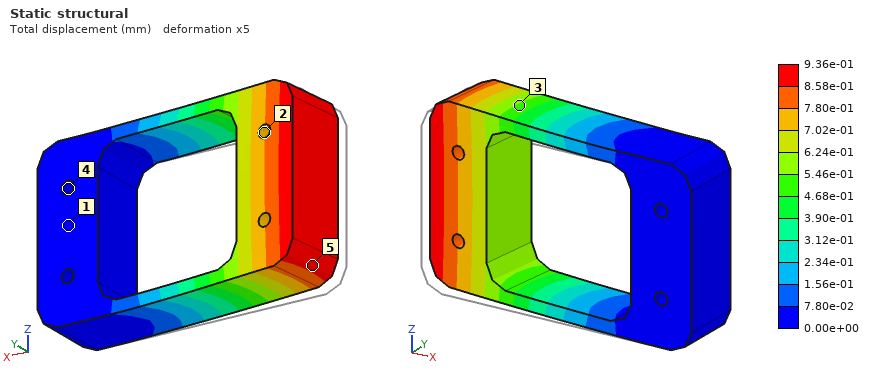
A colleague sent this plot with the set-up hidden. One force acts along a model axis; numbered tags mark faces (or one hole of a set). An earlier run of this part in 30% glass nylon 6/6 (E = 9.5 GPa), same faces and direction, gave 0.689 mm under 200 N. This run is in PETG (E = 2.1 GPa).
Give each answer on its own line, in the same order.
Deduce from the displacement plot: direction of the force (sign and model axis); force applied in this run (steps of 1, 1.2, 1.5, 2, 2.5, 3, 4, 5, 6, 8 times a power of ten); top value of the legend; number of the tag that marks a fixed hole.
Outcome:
+Y
60 N
9.36e-01 mm
4
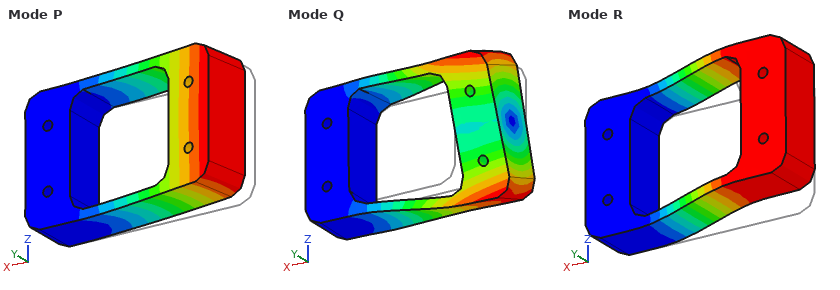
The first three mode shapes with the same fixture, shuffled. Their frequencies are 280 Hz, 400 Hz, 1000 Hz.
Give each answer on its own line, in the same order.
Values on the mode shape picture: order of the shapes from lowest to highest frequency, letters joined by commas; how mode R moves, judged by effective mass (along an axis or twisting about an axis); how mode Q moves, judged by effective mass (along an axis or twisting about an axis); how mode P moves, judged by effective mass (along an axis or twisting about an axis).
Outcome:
R, P, Q
along Z
twisting about X
along Y
